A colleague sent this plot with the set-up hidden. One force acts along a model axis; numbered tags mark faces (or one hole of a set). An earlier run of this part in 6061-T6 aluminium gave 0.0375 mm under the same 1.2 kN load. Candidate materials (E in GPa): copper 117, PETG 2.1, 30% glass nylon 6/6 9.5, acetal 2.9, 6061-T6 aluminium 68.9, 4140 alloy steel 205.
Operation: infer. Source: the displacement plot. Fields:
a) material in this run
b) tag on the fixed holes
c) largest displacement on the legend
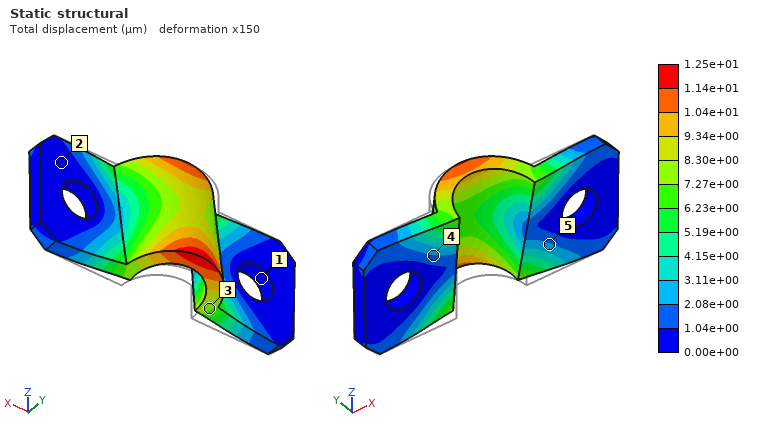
4140 alloy steel
1
1.25e+01 µm
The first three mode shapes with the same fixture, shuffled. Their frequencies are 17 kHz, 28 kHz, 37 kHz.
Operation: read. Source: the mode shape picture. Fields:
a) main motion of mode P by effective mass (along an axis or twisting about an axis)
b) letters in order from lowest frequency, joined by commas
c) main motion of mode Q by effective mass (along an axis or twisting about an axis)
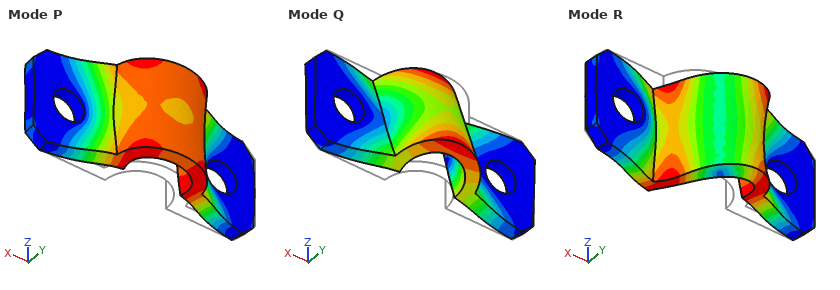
along Y
Q, P, R
along Z
